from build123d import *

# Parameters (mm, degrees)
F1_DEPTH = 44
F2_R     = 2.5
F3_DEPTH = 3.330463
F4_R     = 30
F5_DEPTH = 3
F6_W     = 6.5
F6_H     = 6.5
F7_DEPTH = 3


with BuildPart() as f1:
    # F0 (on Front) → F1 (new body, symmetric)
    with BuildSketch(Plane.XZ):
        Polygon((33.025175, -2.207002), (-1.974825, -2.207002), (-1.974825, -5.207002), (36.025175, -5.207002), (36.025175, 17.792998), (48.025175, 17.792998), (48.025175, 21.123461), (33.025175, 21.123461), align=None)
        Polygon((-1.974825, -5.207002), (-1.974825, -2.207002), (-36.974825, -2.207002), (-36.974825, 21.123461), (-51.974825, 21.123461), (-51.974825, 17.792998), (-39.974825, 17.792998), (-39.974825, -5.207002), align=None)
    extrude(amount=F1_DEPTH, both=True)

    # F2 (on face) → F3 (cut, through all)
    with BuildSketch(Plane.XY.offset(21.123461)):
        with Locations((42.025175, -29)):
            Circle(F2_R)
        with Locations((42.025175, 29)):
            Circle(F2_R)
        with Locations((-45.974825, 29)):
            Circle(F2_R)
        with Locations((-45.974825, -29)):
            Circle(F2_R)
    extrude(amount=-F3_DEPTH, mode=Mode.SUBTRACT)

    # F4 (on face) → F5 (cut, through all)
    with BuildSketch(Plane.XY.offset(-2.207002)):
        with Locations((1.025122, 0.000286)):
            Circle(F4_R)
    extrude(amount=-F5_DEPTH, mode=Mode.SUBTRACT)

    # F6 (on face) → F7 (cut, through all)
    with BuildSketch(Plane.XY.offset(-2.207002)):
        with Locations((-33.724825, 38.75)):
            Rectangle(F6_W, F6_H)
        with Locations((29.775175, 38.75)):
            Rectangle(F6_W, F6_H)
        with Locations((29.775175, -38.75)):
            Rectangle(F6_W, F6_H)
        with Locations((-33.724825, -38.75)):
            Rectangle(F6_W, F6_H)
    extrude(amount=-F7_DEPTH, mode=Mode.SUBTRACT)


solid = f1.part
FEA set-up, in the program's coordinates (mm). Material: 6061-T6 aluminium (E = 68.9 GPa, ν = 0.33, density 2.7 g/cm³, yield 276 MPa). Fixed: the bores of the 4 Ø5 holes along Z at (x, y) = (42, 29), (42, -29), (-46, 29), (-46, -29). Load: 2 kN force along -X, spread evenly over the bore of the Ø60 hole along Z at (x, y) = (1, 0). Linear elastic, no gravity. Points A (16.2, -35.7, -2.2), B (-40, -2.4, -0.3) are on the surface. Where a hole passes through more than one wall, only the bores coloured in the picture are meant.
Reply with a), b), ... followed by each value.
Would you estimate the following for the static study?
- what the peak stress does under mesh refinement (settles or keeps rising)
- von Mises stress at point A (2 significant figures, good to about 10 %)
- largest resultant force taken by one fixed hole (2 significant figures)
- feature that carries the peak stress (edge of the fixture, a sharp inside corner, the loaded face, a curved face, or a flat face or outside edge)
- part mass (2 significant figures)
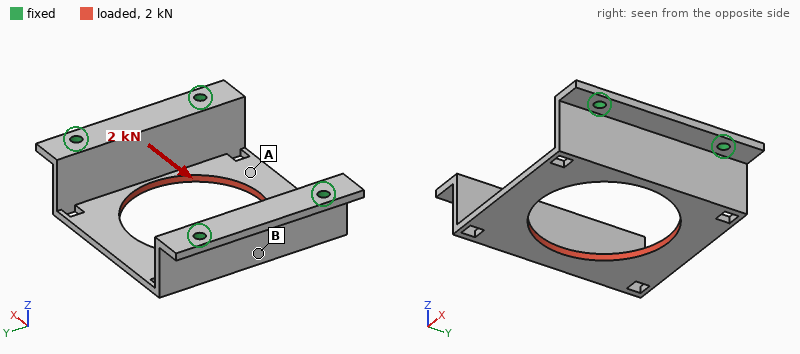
a) keeps rising
b) 69 MPa
c) 520 N
d) edge of the fixture
e) 81 g
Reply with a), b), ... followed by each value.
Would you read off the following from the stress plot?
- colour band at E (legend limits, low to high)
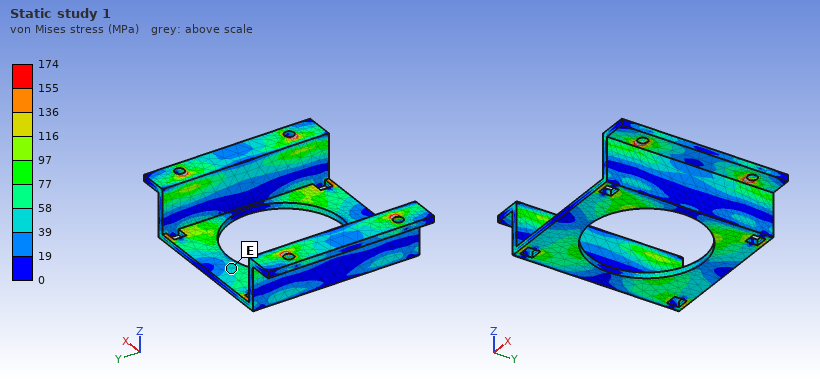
a) 39 to 58 MPa
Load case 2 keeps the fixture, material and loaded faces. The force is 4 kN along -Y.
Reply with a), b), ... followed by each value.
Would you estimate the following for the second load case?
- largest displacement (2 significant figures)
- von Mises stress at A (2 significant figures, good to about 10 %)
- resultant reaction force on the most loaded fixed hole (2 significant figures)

a) 65 µm
b) 20 MPa
c) 1.3 kN
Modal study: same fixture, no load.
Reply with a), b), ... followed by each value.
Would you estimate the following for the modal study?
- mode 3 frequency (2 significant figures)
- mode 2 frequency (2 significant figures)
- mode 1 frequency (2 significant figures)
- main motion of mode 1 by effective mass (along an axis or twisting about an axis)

a) 2600 Hz
b) 2600 Hz
c) 1900 Hz
d) along X
